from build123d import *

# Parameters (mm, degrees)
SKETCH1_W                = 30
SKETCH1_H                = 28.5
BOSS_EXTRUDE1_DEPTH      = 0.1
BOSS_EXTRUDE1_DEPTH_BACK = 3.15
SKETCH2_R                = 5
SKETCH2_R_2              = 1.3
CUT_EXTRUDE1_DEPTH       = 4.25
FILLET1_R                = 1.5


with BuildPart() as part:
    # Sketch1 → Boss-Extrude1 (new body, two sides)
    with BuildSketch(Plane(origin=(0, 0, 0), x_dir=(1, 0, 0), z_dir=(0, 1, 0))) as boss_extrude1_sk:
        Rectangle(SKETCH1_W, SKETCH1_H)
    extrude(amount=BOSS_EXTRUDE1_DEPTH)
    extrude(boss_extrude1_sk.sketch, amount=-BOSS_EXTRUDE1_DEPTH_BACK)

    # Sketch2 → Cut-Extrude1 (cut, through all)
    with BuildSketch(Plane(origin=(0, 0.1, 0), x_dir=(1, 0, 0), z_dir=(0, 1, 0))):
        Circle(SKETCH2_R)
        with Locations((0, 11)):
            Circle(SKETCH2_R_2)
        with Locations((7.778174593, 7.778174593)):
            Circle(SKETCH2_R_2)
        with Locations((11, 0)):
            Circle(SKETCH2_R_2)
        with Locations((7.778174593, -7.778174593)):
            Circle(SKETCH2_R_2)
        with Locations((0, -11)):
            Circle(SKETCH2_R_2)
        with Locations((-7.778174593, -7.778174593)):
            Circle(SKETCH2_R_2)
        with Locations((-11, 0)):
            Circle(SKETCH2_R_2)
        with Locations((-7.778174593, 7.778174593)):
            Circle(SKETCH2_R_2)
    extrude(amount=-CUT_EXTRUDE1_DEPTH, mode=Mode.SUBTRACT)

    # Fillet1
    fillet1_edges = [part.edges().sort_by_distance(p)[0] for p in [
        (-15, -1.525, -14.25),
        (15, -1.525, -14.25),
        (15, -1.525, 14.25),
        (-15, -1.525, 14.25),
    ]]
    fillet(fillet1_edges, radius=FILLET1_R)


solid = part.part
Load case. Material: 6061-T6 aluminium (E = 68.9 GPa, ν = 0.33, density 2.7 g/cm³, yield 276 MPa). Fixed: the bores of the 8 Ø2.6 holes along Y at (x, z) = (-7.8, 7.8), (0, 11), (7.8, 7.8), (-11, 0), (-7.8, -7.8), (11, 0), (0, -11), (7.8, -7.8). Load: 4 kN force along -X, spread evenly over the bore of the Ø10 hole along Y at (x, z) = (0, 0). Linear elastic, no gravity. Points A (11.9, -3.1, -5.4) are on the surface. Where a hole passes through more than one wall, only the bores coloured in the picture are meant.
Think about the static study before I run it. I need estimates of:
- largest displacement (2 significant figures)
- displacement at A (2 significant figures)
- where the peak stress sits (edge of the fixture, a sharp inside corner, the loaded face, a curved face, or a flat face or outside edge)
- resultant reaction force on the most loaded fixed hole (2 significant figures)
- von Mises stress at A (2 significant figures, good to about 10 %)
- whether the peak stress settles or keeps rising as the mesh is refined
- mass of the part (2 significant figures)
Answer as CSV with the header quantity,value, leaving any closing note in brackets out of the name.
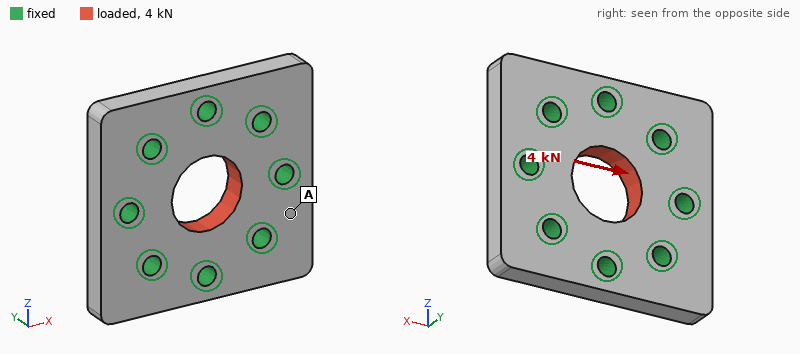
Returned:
quantity,value
largest displacement,3.7 µm
displacement at A,0.68 µm
where the peak stress sits,edge of the fixture
resultant reaction force on the most loaded fixed hole,790 N
von Mises stress at A,8.6 MPa
whether the peak stress settles or keeps rising as the mesh is refined,keeps rising
mass of the part,6.4 g
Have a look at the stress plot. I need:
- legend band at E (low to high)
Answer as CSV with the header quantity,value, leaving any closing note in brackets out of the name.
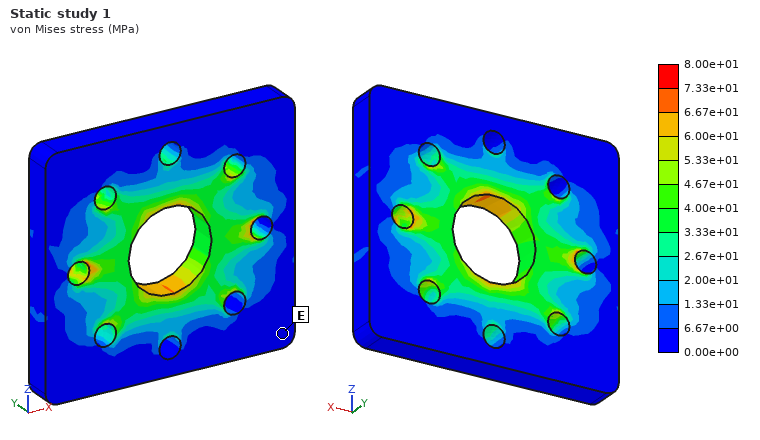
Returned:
quantity,value
legend band at E,0.00e+00 to 6.67e+00 MPa
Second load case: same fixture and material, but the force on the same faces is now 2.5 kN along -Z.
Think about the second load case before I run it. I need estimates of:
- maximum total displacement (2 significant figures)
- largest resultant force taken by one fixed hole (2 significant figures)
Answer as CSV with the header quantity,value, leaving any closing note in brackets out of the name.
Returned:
quantity,value
maximum total displacement,2.3 µm
largest resultant force taken by one fixed hole,490 N
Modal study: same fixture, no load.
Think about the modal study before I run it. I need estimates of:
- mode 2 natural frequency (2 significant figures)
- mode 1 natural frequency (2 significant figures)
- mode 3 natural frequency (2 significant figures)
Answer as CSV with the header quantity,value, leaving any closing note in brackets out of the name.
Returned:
quantity,value
mode 2 natural frequency,46 kHz
mode 1 natural frequency,46 kHz
mode 3 natural frequency,46 kHz
